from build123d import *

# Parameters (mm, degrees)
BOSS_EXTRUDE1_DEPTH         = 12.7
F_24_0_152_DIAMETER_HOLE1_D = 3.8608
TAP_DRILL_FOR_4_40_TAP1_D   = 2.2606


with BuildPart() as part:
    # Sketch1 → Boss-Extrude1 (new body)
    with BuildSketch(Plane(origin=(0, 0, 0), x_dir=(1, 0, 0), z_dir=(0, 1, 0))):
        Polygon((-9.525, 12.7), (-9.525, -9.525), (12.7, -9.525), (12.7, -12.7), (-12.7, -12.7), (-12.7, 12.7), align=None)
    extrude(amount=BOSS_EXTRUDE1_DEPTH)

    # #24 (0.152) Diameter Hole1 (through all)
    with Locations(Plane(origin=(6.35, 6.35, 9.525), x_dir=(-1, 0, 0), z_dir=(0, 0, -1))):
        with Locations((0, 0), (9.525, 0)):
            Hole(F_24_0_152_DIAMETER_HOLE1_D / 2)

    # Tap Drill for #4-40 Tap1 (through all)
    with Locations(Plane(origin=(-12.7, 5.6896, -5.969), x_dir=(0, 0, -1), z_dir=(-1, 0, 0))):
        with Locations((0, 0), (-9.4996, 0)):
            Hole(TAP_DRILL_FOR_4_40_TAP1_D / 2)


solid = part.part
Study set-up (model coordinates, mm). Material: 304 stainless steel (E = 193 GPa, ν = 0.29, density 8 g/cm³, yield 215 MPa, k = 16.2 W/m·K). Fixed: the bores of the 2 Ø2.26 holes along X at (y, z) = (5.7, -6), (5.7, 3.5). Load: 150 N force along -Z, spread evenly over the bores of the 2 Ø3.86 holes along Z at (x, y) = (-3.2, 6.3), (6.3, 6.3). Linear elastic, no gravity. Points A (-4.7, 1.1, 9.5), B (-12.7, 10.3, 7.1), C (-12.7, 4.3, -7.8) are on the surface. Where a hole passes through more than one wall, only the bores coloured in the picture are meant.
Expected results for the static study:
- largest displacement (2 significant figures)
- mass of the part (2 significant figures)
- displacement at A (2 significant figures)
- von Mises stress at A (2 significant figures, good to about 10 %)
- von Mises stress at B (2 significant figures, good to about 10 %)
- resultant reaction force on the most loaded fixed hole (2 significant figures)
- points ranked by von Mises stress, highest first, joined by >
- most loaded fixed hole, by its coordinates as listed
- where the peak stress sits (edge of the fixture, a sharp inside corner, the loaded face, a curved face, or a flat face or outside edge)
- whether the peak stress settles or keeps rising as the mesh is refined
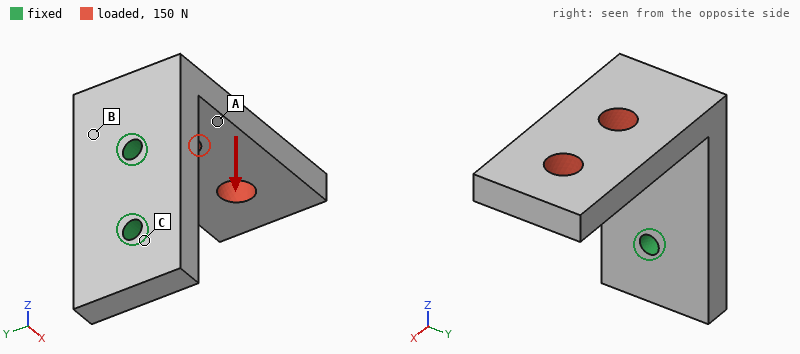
91 µm
15 g
18 µm
56 MPa
75 MPa
140 N
B > A > C
(5.7, 3.5)
edge of the fixture
keeps rising
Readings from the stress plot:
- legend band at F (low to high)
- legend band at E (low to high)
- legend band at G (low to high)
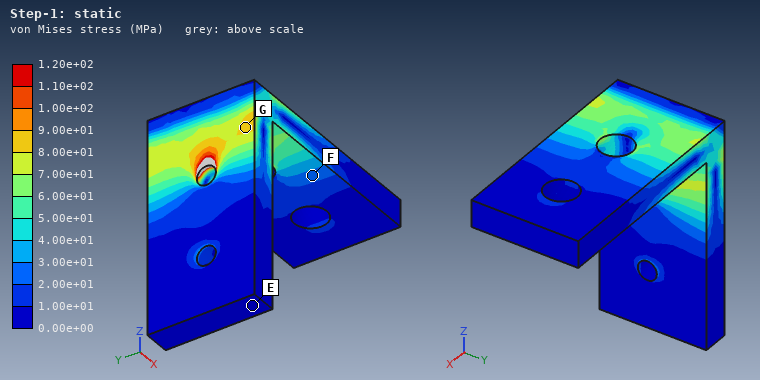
2.00e+01 to 3.00e+01 MPa
0.00e+00 to 1.00e+01 MPa
8.00e+01 to 9.00e+01 MPa
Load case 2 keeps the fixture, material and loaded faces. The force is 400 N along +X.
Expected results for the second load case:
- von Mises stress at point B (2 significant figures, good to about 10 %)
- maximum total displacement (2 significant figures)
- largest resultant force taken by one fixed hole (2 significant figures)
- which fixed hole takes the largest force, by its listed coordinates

58 MPa
49 µm
500 N
(5.7, 3.5)
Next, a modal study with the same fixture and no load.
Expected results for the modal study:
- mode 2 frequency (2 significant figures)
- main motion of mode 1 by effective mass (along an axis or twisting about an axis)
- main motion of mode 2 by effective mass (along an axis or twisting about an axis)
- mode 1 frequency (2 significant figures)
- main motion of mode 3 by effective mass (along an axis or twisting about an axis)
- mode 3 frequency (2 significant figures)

4600 Hz
along Z
along Y
3000 Hz
along X
13 kHz
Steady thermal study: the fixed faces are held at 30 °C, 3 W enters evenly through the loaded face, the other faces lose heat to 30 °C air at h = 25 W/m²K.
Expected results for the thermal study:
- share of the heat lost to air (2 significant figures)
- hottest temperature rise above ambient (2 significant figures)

36 %
68 K
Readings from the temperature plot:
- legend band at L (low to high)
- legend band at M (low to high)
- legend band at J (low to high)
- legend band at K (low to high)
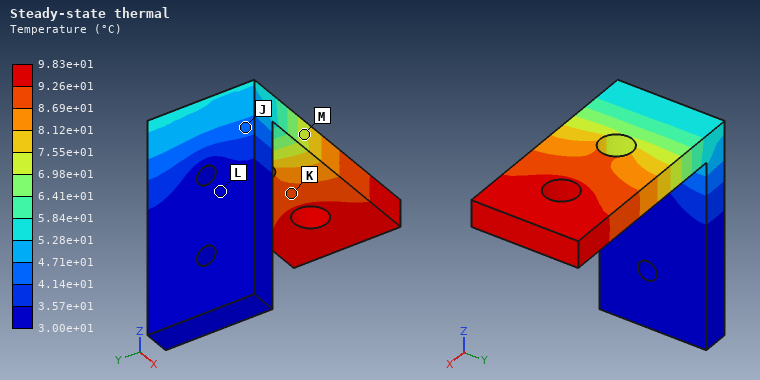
3.00e+01 to 3.57e+01 °C
6.98e+01 to 7.55e+01 °C
4.14e+01 to 4.71e+01 °C
8.69e+01 to 9.26e+01 °C
